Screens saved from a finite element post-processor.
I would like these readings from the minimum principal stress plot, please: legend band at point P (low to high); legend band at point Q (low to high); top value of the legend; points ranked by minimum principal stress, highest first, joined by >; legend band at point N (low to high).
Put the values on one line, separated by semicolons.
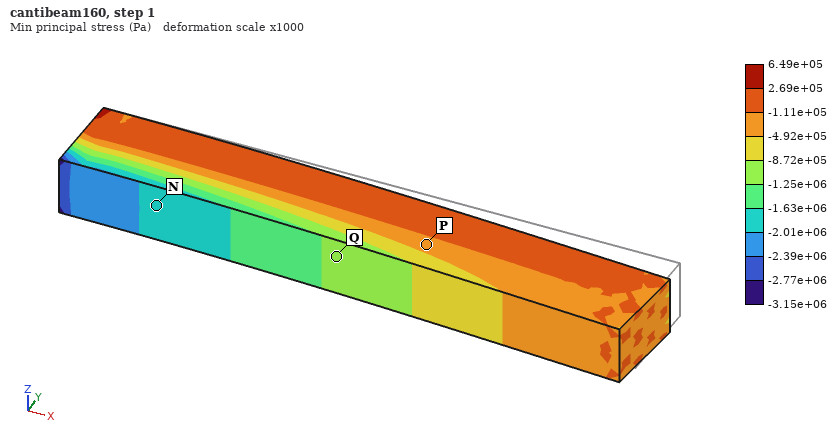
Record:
-4.92e+05 to -1.11e+05 Pa; -1.25e+06 to -8.72e+05 Pa; 6.49e+05 Pa; P > Q > N; -2.01e+06 to -1.63e+06 Pa
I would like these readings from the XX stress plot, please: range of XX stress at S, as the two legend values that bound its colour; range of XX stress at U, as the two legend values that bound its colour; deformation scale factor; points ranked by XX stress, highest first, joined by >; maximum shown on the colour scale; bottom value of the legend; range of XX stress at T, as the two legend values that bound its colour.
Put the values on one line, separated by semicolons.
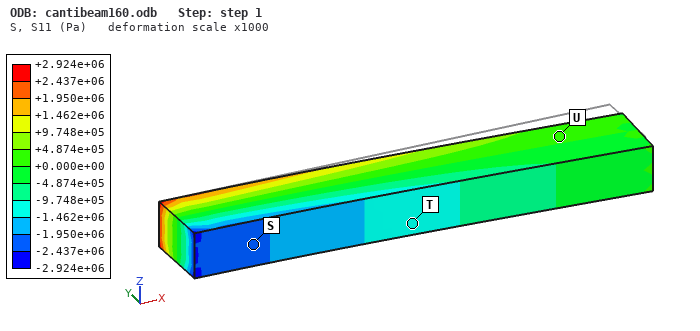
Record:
-2.437e+06 to -1.950e+06 Pa; +0.000e+00 to +4.874e+05 Pa; 1000; U > T > S; +2.924e+06 Pa; -2.924e+06 Pa; -1.462e+06 to -9.748e+05 Pa
